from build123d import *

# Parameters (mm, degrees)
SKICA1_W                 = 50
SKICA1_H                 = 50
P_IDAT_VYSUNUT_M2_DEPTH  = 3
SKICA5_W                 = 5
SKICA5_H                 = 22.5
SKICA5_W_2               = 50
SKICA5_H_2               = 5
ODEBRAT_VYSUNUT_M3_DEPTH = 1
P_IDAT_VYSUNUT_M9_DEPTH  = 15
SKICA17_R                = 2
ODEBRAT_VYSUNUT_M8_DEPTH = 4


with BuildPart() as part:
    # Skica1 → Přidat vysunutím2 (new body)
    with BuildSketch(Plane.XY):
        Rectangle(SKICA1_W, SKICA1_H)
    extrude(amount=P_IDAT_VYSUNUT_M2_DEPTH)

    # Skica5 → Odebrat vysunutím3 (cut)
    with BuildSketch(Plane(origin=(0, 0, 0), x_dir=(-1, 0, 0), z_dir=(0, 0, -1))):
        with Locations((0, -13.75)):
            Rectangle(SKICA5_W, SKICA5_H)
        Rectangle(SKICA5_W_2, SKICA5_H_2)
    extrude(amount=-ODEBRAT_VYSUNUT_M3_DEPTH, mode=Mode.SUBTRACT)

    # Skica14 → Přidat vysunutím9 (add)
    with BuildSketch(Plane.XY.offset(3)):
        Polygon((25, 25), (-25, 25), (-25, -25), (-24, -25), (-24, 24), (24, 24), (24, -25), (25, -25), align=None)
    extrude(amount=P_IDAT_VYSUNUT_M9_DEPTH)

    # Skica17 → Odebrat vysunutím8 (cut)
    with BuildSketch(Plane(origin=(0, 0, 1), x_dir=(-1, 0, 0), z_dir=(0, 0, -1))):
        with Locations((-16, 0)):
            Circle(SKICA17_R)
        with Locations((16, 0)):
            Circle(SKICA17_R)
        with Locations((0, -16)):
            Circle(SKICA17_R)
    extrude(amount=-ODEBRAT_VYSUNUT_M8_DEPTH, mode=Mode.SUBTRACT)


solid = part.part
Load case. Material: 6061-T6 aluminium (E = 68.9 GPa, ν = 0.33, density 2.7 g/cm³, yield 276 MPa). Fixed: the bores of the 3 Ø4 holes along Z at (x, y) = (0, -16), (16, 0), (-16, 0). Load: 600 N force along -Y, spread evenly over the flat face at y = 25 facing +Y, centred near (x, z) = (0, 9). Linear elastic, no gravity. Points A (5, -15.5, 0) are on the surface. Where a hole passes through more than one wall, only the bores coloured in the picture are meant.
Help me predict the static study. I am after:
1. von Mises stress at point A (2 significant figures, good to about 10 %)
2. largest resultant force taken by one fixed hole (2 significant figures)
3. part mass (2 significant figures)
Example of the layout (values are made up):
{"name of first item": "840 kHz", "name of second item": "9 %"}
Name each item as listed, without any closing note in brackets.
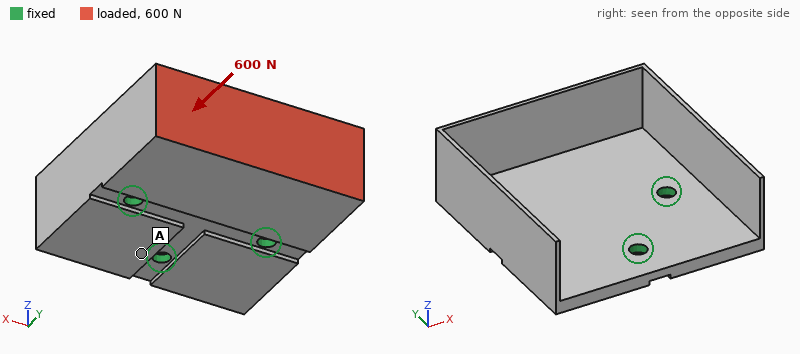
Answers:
{"von Mises stress at point A": "20 MPa", "largest resultant force taken by one fixed hole": "300 N", "part mass": "25 g"}
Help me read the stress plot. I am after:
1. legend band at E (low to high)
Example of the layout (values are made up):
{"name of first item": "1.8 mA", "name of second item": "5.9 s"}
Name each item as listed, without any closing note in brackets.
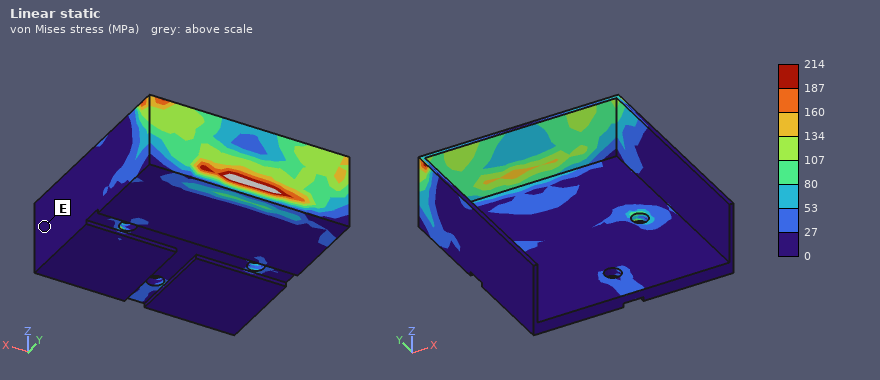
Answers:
{"legend band at E": "0 to 27 MPa"}
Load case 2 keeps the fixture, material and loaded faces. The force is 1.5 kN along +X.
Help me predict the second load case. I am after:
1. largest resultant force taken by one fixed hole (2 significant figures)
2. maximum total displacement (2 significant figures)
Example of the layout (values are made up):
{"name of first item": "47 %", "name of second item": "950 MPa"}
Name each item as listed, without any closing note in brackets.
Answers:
{"largest resultant force taken by one fixed hole": "1.3 kN", "maximum total displacement": "0.32 mm"}
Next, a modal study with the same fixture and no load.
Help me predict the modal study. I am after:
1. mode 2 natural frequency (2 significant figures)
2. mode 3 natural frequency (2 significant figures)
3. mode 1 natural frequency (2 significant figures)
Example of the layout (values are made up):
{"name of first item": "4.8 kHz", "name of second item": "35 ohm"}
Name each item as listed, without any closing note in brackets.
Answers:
{"mode 2 natural frequency": "3400 Hz", "mode 3 natural frequency": "3700 Hz", "mode 1 natural frequency": "2700 Hz"}
